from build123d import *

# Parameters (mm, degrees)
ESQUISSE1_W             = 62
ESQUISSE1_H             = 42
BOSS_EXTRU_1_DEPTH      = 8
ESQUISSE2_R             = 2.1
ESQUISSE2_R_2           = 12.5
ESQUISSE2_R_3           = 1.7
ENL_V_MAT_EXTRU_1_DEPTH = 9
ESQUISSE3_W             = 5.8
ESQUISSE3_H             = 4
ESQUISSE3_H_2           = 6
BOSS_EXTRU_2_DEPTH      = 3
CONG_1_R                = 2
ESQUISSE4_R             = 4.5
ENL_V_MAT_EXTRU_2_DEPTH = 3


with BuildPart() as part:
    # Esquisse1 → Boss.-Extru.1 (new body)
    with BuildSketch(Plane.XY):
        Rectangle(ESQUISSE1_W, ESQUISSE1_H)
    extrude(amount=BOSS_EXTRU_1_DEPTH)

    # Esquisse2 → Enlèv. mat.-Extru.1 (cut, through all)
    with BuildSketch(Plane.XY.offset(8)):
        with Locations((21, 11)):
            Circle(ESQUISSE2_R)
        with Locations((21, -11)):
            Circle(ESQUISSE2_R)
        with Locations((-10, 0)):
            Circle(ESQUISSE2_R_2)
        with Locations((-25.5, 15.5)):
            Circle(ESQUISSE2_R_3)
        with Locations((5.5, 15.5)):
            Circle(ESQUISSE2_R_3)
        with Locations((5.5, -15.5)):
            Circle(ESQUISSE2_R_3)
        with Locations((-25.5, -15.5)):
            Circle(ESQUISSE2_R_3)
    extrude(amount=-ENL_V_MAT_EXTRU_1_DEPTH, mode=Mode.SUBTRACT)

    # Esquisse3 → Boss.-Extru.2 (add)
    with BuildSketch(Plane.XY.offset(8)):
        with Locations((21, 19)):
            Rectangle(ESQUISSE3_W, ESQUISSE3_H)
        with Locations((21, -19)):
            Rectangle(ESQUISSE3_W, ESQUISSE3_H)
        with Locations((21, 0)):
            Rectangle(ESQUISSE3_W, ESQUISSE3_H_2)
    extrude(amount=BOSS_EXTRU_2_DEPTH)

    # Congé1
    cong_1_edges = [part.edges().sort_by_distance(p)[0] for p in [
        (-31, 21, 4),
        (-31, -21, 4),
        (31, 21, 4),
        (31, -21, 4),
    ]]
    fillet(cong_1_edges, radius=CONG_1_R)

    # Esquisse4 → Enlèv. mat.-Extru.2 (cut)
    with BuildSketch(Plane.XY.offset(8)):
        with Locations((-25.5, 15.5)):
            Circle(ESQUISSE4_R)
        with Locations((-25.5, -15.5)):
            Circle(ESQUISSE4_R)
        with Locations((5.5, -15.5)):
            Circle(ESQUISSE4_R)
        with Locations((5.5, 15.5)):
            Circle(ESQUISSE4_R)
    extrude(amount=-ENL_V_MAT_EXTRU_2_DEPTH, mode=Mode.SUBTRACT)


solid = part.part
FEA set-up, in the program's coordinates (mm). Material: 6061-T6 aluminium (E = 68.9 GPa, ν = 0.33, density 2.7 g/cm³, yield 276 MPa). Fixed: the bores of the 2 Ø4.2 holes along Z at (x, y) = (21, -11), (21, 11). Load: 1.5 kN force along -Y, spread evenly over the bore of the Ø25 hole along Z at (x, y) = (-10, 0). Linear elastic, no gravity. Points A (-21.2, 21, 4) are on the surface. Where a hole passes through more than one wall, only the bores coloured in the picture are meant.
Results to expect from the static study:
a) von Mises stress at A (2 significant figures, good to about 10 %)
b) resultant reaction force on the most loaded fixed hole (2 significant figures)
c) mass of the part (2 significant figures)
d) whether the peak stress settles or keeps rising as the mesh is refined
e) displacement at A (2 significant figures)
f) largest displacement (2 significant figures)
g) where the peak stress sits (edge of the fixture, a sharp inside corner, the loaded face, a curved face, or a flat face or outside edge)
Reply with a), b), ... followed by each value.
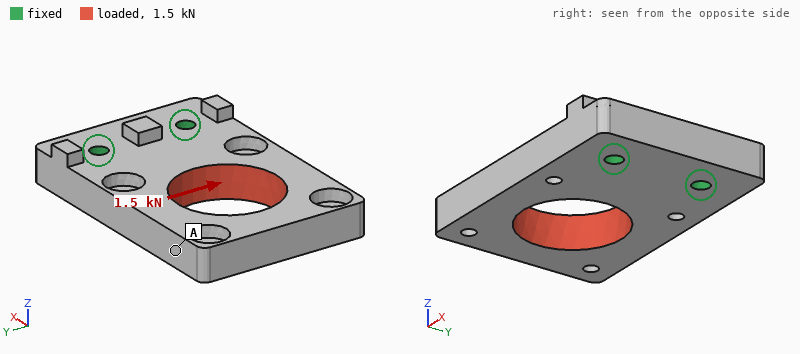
a) 15 MPa
b) 2.0 kN
c) 43 g
d) keeps rising
e) 40 µm
f) 47 µm
g) a sharp inside corner
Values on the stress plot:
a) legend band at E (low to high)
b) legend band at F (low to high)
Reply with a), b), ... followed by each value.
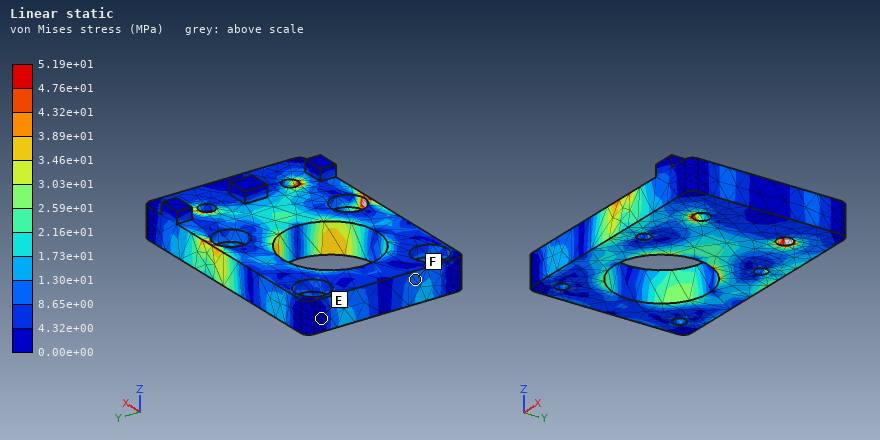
a) 0.00e+00 to 4.32e+00 MPa
b) 8.65e+00 to 1.30e+01 MPa
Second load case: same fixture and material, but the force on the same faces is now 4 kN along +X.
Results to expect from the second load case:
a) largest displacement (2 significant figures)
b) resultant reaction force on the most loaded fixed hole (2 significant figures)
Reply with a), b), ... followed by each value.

a) 33 µm
b) 2.0 kN
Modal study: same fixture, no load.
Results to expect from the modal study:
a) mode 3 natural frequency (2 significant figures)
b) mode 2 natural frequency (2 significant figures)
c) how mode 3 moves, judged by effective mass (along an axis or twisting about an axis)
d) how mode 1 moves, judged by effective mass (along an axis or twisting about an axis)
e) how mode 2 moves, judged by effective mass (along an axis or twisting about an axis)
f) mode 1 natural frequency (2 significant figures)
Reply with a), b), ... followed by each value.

a) 6500 Hz
b) 5100 Hz
c) along Y
d) along Z
e) twisting about X
f) 2200 Hz
